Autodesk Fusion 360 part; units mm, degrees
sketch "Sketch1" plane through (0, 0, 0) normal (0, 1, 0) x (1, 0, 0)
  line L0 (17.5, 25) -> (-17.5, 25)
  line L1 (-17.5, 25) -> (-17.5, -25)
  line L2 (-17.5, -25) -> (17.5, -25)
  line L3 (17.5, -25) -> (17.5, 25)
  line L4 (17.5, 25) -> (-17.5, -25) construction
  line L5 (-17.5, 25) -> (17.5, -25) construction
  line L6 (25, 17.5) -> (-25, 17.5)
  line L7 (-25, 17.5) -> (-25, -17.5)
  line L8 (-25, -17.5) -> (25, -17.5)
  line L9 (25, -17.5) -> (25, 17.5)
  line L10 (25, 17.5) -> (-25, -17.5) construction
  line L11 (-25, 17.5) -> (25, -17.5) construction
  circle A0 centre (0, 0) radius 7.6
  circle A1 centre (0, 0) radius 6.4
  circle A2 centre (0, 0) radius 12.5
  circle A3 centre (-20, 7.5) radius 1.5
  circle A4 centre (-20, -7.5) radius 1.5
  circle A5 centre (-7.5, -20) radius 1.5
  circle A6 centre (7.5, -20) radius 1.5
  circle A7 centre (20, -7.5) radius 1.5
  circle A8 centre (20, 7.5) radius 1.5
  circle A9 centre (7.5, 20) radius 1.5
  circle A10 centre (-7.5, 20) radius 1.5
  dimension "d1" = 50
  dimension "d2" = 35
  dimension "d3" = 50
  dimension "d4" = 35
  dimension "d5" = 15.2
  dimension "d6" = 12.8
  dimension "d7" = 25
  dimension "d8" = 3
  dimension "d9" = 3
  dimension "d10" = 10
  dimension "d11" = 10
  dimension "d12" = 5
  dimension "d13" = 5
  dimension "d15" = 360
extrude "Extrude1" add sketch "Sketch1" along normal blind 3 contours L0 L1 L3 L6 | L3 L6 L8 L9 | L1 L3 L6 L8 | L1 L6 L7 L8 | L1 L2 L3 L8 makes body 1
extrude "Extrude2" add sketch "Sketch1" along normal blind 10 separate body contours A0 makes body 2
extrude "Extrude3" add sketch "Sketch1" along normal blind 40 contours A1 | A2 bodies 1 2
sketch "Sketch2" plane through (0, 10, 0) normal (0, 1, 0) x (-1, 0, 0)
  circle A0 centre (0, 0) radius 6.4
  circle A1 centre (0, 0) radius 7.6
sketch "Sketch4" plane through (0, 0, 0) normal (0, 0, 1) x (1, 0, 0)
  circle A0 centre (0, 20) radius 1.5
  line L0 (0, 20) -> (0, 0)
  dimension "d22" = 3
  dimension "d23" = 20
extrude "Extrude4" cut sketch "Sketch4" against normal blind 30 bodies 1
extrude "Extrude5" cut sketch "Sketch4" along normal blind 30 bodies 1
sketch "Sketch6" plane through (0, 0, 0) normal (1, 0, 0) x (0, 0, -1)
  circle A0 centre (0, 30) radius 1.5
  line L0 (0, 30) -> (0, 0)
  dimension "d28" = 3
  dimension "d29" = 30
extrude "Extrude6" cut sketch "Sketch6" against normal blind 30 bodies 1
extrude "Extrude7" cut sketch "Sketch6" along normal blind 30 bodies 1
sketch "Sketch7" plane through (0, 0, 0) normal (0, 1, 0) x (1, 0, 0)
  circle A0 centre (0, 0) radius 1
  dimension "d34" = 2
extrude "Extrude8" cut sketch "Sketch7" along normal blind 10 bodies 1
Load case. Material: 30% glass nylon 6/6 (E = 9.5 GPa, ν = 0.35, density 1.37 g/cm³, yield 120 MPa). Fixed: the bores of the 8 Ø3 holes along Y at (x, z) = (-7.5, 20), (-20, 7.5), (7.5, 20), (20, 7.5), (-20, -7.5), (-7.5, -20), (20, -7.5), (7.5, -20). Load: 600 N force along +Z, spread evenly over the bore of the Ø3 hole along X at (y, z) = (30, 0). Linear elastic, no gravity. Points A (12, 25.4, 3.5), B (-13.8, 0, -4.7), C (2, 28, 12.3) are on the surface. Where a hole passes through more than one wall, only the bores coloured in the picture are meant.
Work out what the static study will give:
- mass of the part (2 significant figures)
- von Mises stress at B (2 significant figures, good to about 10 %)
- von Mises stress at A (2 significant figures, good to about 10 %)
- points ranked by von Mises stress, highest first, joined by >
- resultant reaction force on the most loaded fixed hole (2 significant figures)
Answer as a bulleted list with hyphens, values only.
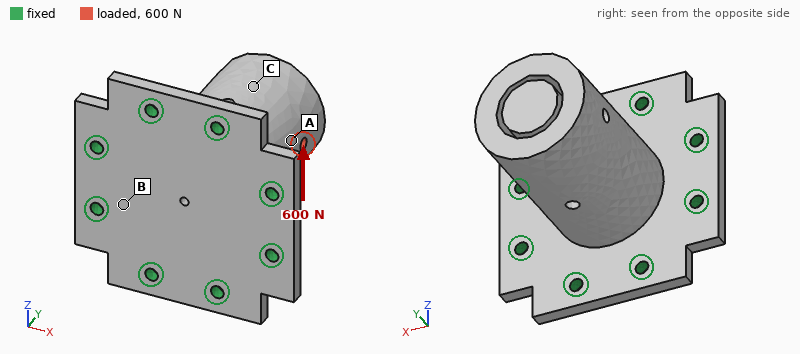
- 31 g
- 15 MPa
- 10 MPa
- B > A > C
- 270 N
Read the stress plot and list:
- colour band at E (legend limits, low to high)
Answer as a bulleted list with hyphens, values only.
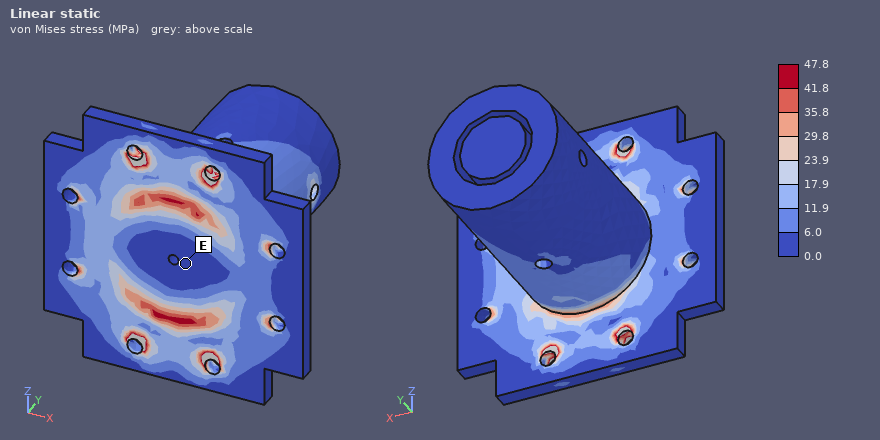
- 0.0 to 6.0 MPa
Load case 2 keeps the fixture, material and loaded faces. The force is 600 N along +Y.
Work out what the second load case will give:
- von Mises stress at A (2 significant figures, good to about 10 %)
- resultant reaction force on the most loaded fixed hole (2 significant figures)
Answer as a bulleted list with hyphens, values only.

- 8.8 MPa
- 160 N
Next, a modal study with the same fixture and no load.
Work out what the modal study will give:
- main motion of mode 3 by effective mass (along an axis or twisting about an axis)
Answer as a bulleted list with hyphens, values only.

- along Y
